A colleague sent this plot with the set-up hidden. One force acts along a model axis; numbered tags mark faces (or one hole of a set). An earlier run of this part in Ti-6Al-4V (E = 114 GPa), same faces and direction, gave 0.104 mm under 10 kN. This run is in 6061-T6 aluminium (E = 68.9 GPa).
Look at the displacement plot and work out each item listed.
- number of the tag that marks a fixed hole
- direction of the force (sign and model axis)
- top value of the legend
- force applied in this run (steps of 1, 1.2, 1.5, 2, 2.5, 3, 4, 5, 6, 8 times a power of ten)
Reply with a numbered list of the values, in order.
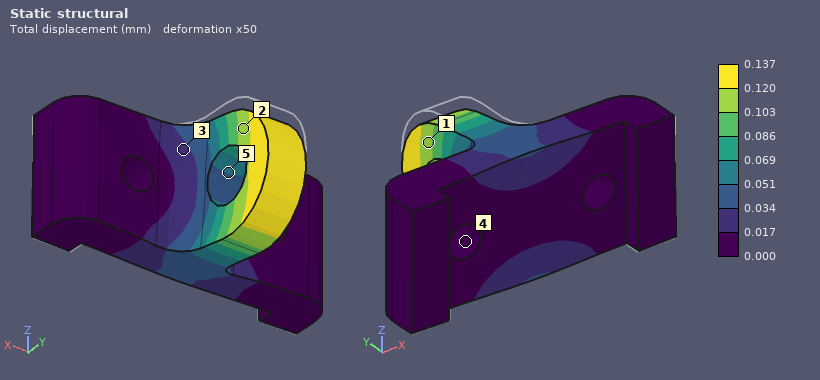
1. 4
2. -Z
3. 0.137 mm
4. 8 kN
